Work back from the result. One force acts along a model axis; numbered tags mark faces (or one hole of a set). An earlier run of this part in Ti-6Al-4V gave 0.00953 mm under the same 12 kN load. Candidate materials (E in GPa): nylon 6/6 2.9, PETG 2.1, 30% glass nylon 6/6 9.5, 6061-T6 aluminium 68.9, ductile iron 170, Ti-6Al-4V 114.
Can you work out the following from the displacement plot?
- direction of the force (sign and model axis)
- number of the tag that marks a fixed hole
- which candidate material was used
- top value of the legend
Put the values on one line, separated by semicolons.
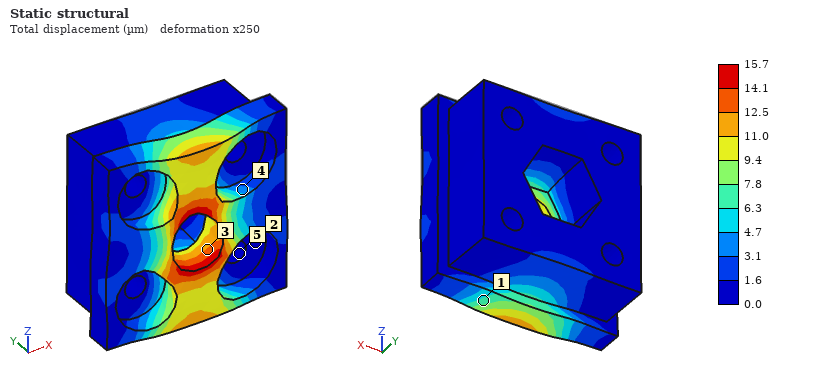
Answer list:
-Z; 5; 6061-T6 aluminium; 15.7 µm
